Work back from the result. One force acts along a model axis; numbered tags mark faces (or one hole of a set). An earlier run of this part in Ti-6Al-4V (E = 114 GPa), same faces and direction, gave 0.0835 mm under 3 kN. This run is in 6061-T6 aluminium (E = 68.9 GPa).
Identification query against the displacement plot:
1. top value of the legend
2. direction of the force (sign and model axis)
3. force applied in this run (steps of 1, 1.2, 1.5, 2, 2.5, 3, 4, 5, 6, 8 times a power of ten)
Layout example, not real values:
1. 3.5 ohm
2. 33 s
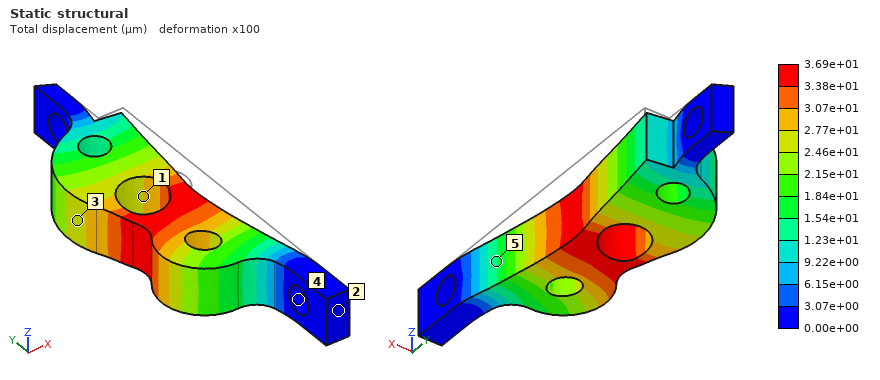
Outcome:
1. 3.69e+01 µm
2. -X
3. 800 N
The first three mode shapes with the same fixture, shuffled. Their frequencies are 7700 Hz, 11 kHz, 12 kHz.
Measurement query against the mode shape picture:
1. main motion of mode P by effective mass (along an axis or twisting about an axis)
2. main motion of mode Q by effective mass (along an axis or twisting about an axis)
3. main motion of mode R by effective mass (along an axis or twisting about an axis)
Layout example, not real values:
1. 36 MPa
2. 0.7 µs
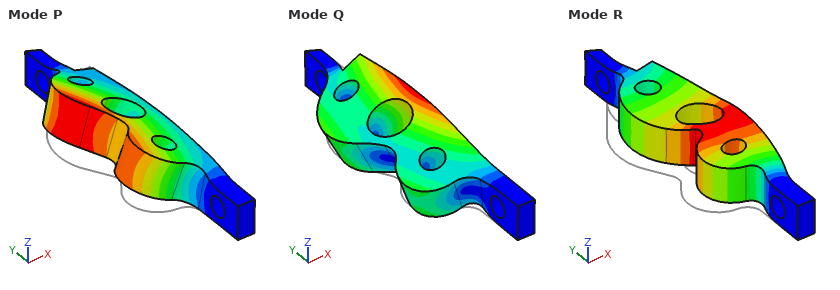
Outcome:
1. along Z
2. along Z
3. along X
